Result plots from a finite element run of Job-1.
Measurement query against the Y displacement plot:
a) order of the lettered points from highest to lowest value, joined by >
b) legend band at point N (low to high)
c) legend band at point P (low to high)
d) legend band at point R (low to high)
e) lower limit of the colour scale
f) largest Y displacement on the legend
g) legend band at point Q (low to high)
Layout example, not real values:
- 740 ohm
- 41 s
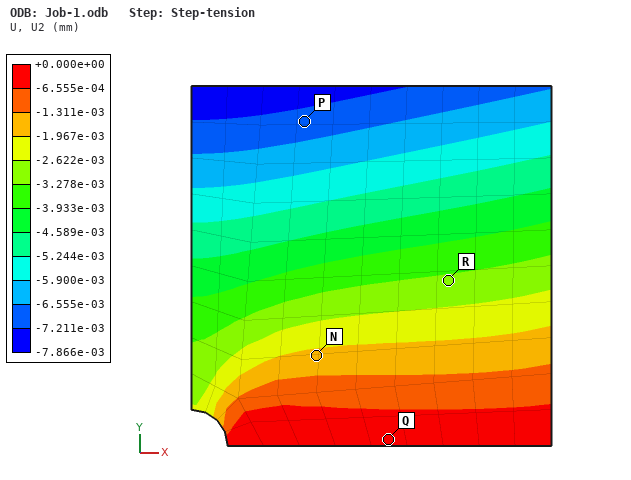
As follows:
- Q > N > R > P
- -1.967e-03 to -1.311e-03 mm
- -7.211e-03 to -6.555e-03 mm
- -3.278e-03 to -2.622e-03 mm
- -7.866e-03 mm
- +0.000e+00 mm
- -6.555e-04 to +0.000e+00 mm
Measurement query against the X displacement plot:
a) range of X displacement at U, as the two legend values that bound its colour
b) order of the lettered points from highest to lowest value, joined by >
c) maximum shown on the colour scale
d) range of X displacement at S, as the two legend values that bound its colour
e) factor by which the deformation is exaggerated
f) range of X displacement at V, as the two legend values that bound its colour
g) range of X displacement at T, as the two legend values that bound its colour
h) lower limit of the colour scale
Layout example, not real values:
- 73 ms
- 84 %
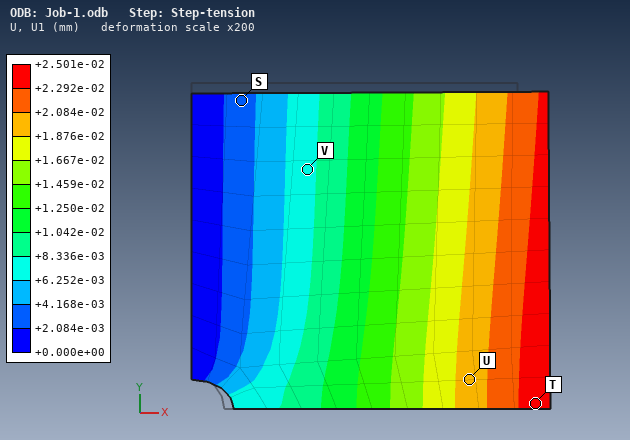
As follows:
- +1.876e-02 to +2.084e-02 mm
- T > U > V > S
- +2.501e-02 mm
- +2.084e-03 to +4.168e-03 mm
- 200
- +6.252e-03 to +8.336e-03 mm
- +2.292e-02 to +2.501e-02 mm
- +0.000e+00 mm
